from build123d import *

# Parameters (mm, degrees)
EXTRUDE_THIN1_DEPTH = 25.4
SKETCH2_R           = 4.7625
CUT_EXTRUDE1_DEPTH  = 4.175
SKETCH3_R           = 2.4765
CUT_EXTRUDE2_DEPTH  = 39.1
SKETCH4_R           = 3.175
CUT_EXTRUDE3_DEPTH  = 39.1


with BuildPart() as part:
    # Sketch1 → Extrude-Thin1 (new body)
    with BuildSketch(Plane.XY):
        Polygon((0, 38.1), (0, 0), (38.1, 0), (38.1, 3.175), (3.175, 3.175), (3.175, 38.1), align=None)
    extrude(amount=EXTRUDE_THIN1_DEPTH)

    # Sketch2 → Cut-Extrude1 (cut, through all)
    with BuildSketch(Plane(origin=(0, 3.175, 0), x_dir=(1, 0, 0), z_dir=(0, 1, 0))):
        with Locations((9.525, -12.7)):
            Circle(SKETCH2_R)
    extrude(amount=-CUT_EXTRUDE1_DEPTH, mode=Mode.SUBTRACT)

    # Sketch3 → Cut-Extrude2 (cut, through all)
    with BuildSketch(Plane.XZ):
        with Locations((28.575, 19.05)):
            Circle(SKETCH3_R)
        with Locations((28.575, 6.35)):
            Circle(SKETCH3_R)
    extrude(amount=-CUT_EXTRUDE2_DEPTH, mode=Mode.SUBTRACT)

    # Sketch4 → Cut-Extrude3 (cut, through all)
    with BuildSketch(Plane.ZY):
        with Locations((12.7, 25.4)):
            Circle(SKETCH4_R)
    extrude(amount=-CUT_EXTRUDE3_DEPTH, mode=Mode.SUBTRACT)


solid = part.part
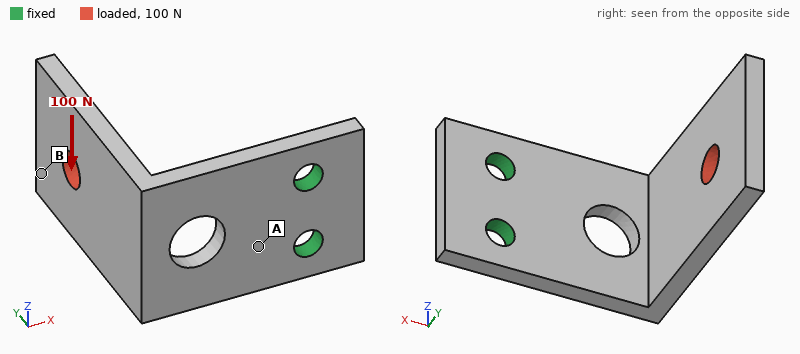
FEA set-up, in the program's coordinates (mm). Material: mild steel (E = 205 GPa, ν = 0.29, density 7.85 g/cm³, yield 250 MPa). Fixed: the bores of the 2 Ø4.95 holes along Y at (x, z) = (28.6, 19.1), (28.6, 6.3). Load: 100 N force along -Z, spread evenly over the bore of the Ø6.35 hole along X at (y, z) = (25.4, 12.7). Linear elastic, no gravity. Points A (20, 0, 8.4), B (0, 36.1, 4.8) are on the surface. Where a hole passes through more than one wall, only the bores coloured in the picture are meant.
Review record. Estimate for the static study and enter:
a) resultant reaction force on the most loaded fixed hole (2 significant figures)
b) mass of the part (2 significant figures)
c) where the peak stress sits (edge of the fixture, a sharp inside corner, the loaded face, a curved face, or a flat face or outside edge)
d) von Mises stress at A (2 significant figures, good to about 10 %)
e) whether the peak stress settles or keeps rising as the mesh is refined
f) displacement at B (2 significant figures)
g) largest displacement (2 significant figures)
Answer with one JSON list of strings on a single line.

["220 N", "43 g", "edge of the fixture", "38 MPa", "keeps rising", "87 µm", "96 µm"]
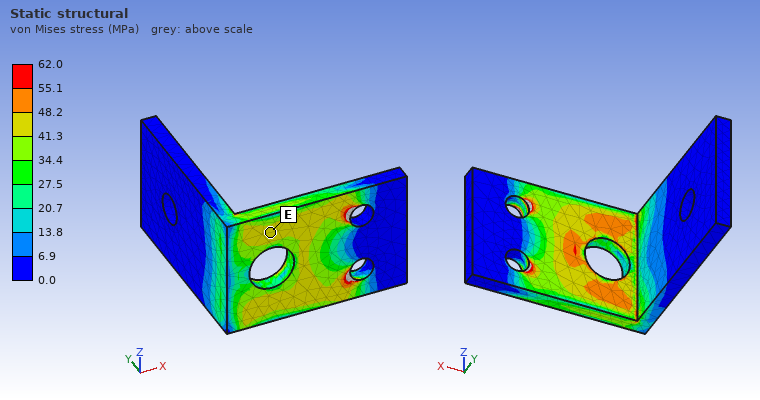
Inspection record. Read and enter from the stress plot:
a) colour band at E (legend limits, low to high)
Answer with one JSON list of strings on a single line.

["41.3 to 48.2 MPa"]
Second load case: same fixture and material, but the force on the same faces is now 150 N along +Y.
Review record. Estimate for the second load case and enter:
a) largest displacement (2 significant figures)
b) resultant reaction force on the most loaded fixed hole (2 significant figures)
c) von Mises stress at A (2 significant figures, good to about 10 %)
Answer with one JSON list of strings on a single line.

["0.16 mm", "75 N", "57 MPa"]
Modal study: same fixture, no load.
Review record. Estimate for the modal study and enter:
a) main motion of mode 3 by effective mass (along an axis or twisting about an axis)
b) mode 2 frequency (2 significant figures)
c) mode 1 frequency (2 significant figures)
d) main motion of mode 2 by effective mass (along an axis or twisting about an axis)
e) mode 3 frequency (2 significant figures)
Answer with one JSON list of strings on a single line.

["along Y", "1500 Hz", "860 Hz", "along Z", "2600 Hz"]
